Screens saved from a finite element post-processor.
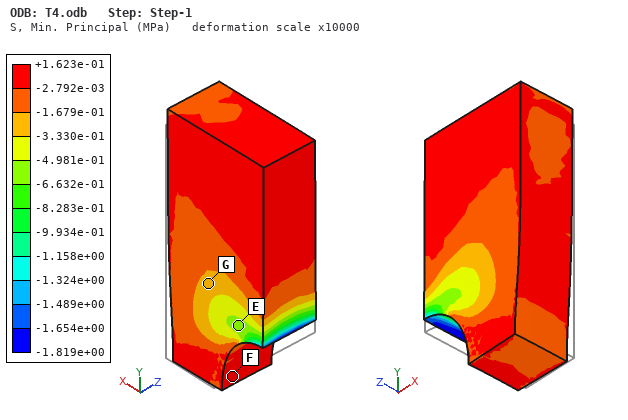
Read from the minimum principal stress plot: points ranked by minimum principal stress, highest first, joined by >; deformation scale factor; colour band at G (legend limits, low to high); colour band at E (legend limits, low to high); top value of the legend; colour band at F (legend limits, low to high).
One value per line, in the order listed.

F > G > E
10000
-3.330e-01 to -1.679e-01 MPa
-6.632e-01 to -4.981e-01 MPa
+1.623e-01 MPa
-2.792e-03 to +1.623e-01 MPa
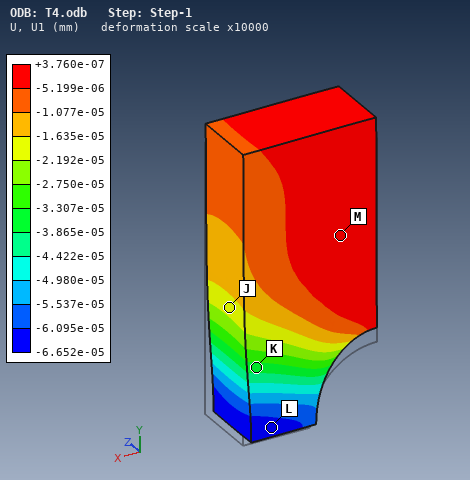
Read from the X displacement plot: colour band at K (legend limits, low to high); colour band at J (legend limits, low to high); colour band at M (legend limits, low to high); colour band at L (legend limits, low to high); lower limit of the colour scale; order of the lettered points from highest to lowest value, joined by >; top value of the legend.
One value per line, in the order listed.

-3.865e-05 to -3.307e-05 mm
-2.192e-05 to -1.635e-05 mm
-5.199e-06 to +3.760e-07 mm
-6.652e-05 to -6.095e-05 mm
-6.652e-05 mm
M > J > K > L
+3.760e-07 mm
